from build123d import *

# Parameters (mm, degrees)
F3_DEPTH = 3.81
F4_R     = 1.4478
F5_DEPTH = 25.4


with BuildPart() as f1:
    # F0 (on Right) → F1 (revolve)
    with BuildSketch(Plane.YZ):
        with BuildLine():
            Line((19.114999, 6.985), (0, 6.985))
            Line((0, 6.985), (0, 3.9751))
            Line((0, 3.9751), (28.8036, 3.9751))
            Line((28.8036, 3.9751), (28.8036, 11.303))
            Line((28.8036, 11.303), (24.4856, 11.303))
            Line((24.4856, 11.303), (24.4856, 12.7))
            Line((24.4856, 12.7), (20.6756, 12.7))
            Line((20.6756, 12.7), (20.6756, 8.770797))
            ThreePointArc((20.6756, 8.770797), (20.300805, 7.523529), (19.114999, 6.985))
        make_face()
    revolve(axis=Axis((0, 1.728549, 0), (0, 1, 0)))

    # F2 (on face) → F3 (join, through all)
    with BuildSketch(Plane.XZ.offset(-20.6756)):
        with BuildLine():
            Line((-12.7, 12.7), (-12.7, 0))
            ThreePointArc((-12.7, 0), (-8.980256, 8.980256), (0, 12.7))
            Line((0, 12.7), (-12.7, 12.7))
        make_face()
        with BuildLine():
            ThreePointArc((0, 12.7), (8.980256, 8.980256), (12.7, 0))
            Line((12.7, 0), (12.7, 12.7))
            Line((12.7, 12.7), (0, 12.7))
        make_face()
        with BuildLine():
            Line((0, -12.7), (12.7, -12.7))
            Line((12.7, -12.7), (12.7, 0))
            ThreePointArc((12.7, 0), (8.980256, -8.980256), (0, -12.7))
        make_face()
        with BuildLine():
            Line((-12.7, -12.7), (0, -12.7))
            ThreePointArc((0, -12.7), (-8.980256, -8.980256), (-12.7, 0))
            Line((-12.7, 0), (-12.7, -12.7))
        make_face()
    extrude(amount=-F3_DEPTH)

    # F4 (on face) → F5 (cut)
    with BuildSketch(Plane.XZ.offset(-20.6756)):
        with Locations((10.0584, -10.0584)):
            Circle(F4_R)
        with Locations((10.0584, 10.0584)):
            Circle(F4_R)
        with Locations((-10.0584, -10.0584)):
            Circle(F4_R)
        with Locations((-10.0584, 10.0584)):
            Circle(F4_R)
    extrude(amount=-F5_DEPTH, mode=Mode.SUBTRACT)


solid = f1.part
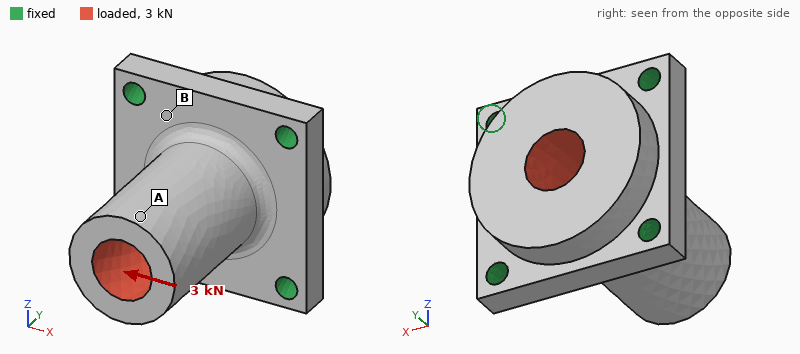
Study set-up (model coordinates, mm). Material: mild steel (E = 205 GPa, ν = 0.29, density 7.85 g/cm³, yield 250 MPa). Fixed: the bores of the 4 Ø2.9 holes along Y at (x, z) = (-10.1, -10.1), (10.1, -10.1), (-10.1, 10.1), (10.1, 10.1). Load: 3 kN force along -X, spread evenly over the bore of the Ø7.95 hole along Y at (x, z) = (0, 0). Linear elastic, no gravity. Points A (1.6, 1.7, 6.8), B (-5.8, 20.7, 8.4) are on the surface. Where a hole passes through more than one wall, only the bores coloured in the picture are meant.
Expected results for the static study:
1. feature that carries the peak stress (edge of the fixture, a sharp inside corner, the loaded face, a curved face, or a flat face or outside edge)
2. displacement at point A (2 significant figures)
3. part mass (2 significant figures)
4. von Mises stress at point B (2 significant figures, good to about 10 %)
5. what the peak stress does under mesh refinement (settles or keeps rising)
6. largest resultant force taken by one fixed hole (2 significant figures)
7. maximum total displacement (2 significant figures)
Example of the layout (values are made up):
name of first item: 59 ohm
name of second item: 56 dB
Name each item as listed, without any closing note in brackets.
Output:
feature that carries the peak stress: edge of the fixture
displacement at point A: 20 µm
part mass: 46 g
von Mises stress at point B: 57 MPa
what the peak stress does under mesh refinement: keeps rising
largest resultant force taken by one fixed hole: 1.0 kN
maximum total displacement: 23 µm
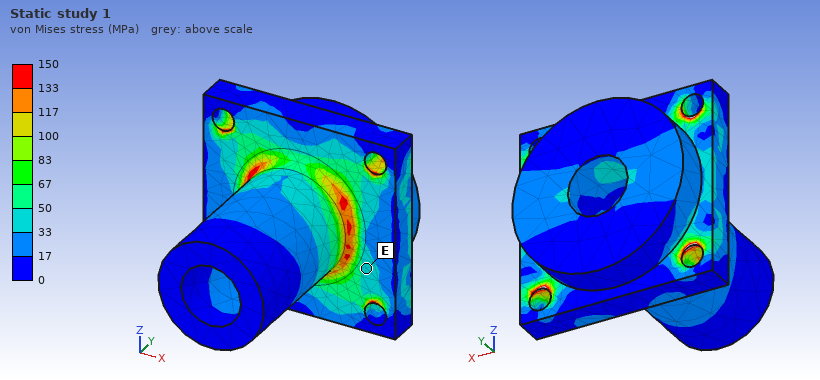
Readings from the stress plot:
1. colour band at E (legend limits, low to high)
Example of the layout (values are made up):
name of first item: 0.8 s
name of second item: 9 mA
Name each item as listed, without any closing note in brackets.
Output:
colour band at E: 33 to 50 MPa
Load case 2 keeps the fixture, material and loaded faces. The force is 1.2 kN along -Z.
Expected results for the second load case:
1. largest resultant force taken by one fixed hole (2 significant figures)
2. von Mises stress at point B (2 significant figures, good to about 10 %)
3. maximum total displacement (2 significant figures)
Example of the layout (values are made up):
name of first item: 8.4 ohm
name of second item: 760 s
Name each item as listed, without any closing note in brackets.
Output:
largest resultant force taken by one fixed hole: 410 N
von Mises stress at point B: 19 MPa
maximum total displacement: 9.1 µm
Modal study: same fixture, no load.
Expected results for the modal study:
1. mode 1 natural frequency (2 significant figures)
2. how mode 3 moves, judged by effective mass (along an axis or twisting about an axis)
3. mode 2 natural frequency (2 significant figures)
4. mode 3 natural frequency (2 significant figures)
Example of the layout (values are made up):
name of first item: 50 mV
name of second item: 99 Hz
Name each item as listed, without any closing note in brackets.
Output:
mode 1 natural frequency: 14 kHz
how mode 3 moves, judged by effective mass: along Y
mode 2 natural frequency: 14 kHz
mode 3 natural frequency: 26 kHz
